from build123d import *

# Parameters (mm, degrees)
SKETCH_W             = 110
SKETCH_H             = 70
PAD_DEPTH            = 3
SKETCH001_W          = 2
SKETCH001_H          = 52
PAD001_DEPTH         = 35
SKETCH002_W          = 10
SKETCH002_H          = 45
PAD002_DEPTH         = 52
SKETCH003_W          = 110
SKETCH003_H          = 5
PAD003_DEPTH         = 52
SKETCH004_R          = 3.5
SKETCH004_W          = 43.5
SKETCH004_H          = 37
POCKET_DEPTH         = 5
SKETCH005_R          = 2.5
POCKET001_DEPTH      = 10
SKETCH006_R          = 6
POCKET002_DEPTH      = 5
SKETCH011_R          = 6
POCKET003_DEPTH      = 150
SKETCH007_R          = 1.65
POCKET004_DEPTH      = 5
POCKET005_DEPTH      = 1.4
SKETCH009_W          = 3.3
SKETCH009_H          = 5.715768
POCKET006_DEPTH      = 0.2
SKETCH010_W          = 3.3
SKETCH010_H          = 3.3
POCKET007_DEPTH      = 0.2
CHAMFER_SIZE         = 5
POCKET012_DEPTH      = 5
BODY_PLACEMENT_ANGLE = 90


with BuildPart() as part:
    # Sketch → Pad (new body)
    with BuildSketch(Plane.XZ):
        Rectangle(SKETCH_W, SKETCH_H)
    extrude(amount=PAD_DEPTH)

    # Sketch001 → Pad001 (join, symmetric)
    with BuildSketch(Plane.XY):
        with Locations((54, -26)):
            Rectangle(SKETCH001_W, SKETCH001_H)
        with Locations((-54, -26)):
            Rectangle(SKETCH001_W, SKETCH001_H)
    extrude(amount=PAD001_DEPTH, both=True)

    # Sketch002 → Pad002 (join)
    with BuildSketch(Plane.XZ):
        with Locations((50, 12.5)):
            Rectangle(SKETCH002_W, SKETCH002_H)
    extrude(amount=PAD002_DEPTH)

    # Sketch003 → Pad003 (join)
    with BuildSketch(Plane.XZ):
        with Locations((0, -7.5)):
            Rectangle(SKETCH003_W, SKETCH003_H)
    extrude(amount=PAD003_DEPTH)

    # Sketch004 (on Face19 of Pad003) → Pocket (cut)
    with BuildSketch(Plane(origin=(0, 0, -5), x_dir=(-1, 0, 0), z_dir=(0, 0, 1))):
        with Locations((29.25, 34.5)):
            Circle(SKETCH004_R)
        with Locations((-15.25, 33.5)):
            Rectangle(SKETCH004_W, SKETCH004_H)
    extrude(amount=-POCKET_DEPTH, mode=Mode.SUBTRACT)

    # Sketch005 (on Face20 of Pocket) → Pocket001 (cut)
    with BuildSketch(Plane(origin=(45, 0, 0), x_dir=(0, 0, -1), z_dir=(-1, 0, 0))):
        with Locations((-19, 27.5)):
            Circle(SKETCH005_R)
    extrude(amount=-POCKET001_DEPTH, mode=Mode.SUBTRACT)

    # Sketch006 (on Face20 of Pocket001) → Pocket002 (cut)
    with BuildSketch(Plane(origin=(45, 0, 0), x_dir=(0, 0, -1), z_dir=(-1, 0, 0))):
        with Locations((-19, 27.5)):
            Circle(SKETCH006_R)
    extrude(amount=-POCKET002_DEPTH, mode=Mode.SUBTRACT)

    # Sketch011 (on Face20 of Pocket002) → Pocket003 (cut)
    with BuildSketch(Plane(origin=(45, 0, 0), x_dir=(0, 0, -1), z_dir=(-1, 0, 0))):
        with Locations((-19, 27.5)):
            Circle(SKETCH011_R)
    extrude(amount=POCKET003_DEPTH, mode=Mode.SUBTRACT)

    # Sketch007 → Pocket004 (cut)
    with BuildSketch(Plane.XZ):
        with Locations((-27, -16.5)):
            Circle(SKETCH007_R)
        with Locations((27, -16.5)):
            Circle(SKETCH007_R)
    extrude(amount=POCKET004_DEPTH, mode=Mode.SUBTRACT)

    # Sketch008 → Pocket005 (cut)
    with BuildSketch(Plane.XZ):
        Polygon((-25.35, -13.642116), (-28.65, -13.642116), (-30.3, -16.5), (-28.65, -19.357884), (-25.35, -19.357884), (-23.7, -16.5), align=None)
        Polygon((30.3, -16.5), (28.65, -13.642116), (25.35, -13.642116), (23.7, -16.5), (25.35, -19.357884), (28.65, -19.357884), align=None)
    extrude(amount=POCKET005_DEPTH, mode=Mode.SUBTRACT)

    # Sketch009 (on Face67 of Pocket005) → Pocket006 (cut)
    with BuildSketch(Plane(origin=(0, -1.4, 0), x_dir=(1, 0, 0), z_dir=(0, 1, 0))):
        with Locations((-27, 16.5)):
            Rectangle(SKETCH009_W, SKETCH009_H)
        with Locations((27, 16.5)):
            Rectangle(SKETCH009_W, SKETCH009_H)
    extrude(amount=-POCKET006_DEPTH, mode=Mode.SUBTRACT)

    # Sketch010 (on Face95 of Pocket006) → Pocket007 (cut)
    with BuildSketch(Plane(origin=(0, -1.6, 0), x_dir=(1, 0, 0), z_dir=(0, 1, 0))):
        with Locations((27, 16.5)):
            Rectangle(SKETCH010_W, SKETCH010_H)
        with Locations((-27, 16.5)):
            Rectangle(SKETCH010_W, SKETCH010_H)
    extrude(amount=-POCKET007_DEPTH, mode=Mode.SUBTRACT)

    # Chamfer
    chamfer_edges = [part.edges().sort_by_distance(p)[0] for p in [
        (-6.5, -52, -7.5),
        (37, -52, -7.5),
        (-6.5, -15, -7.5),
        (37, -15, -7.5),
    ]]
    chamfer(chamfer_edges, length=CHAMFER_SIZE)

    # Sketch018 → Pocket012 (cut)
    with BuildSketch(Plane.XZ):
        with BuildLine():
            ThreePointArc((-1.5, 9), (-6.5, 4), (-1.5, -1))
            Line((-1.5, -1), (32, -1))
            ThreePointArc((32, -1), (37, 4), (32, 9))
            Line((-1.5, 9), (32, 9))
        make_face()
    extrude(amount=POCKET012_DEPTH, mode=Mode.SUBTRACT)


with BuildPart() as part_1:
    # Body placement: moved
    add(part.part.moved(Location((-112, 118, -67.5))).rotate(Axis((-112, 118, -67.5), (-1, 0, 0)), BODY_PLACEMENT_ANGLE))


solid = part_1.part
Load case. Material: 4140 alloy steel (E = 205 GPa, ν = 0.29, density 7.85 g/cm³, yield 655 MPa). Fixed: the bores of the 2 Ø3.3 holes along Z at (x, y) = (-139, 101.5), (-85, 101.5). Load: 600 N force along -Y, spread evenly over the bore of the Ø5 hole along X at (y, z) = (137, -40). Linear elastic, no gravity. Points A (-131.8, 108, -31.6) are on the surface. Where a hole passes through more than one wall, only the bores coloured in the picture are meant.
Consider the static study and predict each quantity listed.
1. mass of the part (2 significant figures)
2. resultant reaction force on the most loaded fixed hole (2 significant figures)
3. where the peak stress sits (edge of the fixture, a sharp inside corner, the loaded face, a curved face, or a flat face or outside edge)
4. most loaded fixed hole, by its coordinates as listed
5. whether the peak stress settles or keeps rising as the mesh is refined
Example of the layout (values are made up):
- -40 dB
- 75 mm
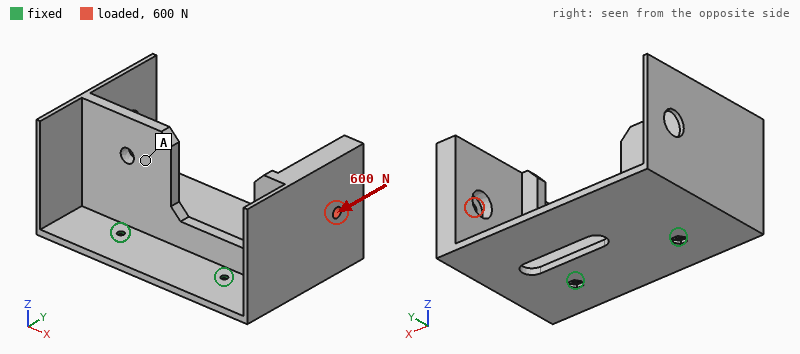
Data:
- 530 g
- 880 N
- edge of the fixture
- (-85, 101.5)
- keeps rising
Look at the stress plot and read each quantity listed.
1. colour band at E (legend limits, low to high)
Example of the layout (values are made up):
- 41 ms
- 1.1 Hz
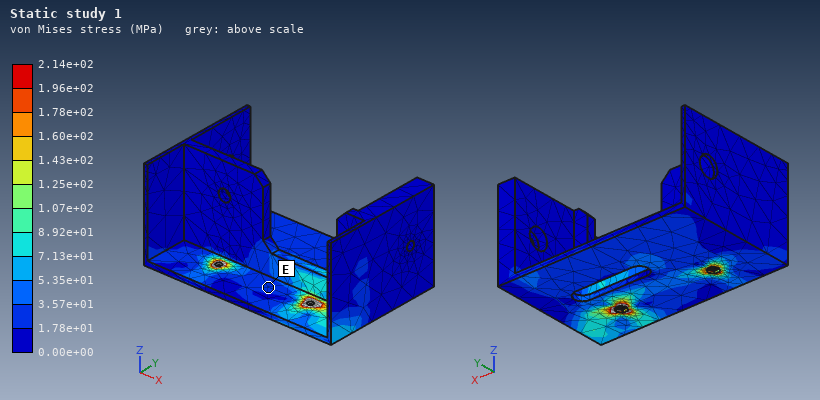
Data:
- 1.78e+01 to 3.57e+01 MPa
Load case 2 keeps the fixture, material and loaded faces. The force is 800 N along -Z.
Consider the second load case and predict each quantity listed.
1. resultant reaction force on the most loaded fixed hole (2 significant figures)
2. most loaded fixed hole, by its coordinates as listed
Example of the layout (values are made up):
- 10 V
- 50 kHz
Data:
- 1.2 kN
- (-85, 101.5)
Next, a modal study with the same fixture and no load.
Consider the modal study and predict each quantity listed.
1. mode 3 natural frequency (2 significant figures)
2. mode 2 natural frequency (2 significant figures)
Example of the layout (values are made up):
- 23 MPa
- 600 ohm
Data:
- 1200 Hz
- 550 Hz
